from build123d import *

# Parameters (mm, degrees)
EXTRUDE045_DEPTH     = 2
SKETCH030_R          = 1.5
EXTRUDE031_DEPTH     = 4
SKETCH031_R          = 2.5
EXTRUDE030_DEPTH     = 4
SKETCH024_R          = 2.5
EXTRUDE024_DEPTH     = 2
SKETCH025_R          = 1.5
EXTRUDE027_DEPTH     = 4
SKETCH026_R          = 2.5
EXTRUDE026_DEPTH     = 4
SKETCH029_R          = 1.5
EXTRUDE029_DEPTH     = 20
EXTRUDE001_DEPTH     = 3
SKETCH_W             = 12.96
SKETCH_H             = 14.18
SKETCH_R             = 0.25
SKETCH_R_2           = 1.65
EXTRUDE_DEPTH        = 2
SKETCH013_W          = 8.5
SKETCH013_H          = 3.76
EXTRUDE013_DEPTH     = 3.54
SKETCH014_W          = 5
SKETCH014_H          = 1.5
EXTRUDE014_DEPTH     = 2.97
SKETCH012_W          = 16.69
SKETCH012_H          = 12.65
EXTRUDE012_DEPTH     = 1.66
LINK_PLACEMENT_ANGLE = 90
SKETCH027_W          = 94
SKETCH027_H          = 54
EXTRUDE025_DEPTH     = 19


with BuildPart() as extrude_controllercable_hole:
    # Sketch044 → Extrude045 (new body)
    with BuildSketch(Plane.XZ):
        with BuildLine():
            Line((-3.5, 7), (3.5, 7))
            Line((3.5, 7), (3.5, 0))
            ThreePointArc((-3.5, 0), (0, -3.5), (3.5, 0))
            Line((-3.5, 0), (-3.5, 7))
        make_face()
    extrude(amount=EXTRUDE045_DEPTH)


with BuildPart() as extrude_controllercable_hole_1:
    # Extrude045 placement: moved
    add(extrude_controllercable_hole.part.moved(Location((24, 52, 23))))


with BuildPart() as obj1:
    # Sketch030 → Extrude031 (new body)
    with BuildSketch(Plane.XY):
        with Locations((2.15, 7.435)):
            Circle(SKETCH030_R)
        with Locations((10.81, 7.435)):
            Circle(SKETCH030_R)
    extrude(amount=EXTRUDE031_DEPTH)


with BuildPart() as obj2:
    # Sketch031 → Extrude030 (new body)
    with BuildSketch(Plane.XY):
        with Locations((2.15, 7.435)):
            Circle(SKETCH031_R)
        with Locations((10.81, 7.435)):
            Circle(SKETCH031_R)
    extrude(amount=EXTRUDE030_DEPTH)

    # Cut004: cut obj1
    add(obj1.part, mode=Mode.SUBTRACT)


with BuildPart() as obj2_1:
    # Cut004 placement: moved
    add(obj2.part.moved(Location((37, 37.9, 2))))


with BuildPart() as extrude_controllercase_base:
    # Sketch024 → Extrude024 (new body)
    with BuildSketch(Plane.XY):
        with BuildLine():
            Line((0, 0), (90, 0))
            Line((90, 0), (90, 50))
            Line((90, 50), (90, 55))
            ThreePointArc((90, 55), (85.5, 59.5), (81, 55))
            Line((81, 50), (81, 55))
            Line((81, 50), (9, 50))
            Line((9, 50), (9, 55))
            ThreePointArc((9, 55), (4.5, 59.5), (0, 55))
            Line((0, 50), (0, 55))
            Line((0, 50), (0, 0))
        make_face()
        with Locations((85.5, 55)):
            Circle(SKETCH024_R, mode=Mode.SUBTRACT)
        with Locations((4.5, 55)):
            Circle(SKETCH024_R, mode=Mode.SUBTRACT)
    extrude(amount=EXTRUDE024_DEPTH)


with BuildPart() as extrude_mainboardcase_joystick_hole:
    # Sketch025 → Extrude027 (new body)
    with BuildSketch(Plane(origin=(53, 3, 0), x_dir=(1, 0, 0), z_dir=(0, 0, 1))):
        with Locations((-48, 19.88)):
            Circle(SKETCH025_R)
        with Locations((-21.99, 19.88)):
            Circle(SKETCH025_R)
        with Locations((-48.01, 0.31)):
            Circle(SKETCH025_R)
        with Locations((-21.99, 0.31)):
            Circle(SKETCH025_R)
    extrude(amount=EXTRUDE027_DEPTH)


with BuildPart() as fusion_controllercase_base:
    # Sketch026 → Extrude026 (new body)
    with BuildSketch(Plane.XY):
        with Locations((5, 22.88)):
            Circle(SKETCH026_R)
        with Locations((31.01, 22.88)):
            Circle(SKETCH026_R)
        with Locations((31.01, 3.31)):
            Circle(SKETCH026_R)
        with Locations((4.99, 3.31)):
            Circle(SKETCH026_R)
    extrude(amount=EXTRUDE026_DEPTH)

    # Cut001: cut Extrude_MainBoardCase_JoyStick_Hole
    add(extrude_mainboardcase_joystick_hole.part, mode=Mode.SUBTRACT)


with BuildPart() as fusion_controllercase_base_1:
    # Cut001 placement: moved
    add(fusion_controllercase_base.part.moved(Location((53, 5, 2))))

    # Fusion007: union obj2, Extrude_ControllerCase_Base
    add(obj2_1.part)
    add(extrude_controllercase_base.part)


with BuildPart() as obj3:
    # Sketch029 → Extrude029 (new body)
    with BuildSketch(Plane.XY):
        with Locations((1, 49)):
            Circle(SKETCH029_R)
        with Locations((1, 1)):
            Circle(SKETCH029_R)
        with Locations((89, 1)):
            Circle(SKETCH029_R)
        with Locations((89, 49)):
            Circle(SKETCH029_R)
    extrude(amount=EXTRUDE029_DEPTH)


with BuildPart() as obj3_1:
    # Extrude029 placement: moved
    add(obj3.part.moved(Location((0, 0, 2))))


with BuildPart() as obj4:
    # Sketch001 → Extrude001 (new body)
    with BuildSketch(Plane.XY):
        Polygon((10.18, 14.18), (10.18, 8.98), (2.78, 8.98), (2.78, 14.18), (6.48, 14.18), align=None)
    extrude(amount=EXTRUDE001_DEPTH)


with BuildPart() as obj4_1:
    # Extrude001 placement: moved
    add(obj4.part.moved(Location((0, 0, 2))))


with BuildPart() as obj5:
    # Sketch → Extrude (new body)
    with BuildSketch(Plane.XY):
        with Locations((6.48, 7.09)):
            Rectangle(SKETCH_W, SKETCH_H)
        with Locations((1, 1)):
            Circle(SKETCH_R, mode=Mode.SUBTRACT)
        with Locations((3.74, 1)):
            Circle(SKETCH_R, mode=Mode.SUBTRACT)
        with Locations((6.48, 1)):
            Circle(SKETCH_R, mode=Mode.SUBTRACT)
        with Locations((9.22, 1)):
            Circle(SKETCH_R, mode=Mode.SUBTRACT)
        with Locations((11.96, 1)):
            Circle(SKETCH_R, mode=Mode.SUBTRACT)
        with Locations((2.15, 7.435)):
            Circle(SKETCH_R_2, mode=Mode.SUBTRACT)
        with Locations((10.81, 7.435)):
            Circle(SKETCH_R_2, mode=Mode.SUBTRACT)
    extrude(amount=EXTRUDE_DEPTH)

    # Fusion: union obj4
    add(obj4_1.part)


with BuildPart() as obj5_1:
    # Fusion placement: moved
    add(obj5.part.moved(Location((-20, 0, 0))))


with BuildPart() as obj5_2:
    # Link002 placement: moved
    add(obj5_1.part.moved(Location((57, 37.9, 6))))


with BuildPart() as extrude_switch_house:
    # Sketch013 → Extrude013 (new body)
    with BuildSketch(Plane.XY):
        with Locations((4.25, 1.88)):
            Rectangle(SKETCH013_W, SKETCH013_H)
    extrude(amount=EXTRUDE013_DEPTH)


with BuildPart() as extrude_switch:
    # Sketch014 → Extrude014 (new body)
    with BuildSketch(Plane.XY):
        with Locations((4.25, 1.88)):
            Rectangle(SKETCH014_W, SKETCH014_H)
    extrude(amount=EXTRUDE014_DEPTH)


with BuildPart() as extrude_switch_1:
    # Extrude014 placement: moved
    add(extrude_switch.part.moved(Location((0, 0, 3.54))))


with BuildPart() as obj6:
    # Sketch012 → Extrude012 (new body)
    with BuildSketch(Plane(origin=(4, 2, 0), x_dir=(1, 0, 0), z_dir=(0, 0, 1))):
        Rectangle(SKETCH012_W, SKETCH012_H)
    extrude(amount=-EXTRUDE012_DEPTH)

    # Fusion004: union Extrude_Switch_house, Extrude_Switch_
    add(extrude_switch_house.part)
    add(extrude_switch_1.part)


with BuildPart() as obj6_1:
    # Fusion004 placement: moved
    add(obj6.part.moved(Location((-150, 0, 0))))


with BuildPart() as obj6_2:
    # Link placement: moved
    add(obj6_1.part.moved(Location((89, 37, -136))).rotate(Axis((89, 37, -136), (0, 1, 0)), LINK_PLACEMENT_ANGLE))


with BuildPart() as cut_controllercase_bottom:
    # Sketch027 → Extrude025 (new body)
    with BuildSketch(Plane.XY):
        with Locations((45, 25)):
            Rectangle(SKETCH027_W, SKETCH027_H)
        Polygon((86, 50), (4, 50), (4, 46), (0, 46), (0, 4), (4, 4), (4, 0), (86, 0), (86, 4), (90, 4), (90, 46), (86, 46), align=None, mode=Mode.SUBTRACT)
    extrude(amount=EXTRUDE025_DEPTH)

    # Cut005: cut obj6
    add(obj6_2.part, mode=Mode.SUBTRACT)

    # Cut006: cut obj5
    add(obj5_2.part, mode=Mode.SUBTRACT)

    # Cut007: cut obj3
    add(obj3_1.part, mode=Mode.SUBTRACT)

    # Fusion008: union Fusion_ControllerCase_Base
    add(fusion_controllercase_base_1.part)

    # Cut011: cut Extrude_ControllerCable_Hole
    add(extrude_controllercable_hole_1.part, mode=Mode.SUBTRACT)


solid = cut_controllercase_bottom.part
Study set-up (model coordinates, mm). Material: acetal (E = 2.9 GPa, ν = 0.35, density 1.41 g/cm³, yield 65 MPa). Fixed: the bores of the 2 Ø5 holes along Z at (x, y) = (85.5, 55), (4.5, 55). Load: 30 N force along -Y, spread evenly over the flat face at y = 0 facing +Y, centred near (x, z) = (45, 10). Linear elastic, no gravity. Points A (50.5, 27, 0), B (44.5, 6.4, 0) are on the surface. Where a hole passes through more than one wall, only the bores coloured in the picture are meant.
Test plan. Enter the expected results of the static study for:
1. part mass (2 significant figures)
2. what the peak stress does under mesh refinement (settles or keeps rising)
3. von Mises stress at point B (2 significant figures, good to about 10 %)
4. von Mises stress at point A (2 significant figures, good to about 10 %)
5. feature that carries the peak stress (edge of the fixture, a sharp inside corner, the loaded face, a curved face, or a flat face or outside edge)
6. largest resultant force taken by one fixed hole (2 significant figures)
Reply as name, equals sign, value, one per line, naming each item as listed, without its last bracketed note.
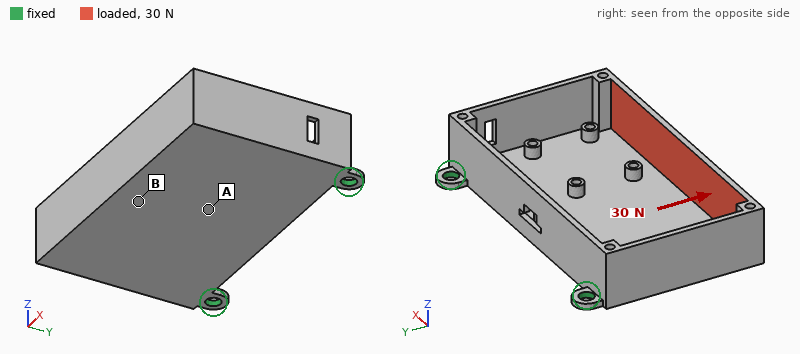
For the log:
part mass = 29 g
what the peak stress does under mesh refinement = keeps rising
von Mises stress at point B = 2.0 MPa
von Mises stress at point A = 0.63 MPa
feature that carries the peak stress = edge of the fixture
largest resultant force taken by one fixed hole = 15 N
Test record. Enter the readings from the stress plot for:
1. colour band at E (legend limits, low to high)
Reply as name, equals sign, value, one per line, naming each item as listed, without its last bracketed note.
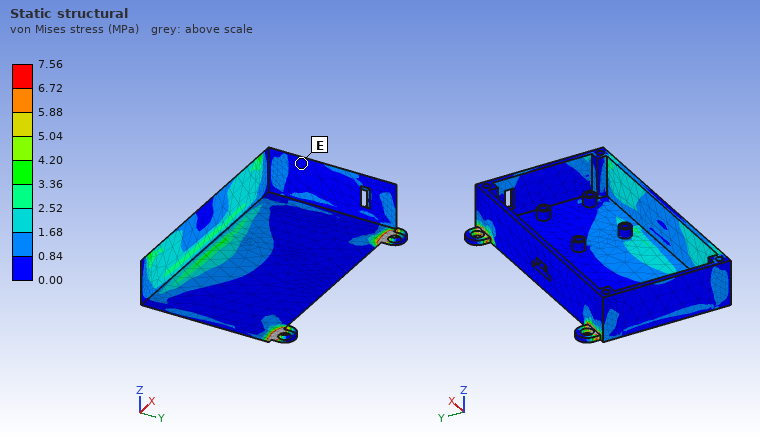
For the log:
colour band at E = 0.00 to 0.84 MPa
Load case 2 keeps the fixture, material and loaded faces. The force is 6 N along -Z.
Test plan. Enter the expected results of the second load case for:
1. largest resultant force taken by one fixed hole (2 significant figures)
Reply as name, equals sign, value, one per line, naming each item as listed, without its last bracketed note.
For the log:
largest resultant force taken by one fixed hole = 3.1 N
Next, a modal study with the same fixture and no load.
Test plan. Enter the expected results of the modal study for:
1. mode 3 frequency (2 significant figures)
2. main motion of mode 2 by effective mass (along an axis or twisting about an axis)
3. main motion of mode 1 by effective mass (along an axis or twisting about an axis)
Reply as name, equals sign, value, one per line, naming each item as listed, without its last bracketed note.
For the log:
mode 3 frequency = 770 Hz
main motion of mode 2 by effective mass = twisting about Y
main motion of mode 1 by effective mass = along Z
